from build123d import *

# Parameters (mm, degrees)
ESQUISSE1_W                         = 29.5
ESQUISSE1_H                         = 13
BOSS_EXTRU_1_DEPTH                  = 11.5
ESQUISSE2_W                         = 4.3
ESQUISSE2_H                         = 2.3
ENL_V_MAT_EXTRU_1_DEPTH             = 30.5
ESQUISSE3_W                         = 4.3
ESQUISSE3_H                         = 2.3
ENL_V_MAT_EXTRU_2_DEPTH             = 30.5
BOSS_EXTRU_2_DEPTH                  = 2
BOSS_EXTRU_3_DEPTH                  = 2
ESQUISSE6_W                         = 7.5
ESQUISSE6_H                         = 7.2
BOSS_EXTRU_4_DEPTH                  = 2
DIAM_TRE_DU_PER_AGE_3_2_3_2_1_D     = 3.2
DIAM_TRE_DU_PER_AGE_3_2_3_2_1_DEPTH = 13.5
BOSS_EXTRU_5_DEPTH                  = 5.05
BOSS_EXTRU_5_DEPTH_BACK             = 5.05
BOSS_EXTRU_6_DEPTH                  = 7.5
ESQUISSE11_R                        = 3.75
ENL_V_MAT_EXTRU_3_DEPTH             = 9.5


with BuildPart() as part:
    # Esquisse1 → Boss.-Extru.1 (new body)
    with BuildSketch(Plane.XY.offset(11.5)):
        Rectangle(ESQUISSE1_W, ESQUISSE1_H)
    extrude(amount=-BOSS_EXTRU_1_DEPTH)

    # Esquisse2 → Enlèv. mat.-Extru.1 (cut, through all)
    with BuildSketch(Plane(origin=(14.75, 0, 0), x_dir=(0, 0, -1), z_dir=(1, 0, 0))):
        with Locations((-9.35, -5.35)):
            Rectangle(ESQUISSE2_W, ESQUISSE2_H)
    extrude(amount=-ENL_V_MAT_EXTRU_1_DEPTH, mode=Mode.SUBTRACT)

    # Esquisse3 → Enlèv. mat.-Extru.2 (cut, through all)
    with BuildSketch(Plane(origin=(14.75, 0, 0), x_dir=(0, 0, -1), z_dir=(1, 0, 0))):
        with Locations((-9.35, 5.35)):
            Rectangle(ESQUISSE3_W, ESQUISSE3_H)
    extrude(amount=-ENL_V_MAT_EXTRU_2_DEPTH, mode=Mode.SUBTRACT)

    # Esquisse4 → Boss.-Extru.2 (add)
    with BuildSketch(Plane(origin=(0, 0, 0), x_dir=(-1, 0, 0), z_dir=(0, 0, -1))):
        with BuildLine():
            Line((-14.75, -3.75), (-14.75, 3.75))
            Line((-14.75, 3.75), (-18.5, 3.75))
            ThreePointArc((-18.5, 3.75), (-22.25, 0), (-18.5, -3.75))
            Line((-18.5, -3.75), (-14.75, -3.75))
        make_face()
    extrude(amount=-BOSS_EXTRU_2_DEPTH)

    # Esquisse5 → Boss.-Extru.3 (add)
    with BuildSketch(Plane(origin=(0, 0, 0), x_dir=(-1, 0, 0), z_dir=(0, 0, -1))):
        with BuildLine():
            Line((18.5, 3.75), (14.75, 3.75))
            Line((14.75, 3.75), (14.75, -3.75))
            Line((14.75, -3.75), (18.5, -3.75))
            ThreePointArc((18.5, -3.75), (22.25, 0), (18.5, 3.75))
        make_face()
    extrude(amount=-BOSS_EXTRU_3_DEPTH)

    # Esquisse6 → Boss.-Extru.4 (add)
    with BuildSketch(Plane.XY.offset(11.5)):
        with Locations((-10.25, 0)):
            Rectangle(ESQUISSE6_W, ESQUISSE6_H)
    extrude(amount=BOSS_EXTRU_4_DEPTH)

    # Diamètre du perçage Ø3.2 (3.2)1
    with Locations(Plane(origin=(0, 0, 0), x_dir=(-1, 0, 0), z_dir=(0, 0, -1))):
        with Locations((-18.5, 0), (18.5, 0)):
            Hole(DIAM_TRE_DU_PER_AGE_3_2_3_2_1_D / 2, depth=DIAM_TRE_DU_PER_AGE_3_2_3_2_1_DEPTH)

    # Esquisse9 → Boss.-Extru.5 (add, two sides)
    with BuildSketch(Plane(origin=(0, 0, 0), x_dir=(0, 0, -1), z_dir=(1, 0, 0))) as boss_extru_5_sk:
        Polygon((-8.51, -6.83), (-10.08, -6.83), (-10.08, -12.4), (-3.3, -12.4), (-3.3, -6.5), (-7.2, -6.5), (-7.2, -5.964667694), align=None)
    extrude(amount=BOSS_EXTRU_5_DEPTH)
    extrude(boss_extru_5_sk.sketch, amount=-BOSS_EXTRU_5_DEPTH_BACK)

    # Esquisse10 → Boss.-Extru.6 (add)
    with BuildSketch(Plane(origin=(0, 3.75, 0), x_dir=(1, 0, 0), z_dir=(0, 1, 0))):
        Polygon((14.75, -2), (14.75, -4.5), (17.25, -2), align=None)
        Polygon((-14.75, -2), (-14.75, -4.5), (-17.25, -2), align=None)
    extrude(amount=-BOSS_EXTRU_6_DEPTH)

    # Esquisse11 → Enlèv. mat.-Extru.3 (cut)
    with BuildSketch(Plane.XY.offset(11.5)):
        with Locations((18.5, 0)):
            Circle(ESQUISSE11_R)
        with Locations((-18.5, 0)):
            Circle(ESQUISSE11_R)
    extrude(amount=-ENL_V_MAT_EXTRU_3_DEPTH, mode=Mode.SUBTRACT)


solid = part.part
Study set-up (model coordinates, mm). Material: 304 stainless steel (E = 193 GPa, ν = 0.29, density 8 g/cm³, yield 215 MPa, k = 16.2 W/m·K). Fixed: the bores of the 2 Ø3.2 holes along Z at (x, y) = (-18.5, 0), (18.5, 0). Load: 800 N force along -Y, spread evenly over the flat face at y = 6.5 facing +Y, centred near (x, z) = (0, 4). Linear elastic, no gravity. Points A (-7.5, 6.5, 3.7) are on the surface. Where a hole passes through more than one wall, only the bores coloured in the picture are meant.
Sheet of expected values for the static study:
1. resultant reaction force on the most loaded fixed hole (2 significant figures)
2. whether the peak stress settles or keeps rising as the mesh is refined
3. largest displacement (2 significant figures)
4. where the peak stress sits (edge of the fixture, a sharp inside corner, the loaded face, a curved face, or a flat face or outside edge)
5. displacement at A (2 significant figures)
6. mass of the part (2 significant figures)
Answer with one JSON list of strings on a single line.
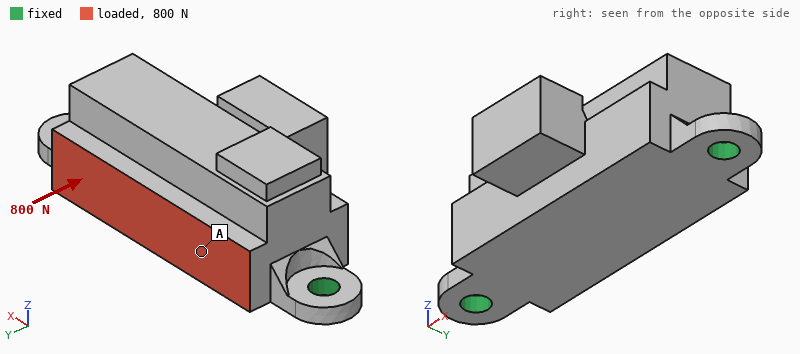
["400 N", "keeps rising", "21 µm", "edge of the fixture", "10 µm", "36 g"]
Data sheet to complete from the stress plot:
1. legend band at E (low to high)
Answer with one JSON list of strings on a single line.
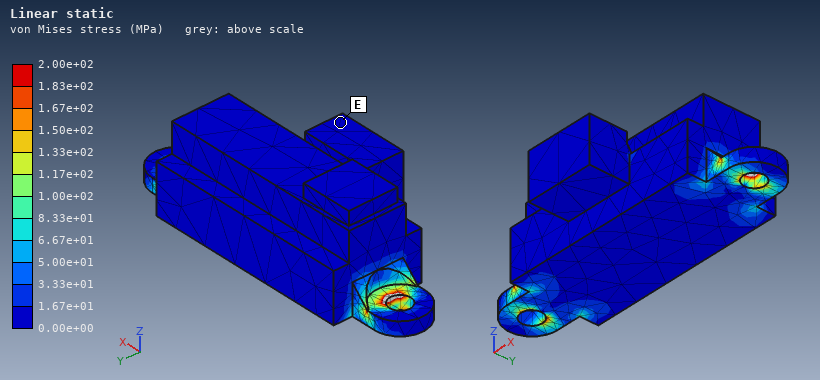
["0.00e+00 to 1.67e+01 MPa"]
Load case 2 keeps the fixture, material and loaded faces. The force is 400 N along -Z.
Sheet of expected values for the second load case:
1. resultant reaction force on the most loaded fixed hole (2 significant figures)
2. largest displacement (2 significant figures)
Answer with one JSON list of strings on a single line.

["250 N", "23 µm"]
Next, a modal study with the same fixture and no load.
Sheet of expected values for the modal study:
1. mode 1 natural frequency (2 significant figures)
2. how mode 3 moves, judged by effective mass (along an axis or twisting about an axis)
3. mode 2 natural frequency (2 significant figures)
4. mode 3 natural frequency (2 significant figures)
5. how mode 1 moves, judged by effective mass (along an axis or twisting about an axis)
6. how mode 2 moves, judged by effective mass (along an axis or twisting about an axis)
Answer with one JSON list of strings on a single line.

["4700 Hz", "along Y", "13 kHz", "18 kHz", "along Y", "along Z"]
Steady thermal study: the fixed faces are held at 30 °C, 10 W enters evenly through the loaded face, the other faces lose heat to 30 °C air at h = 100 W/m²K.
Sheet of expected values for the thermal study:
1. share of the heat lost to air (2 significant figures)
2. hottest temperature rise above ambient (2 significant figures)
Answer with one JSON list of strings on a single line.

["61 %", "52 K"]
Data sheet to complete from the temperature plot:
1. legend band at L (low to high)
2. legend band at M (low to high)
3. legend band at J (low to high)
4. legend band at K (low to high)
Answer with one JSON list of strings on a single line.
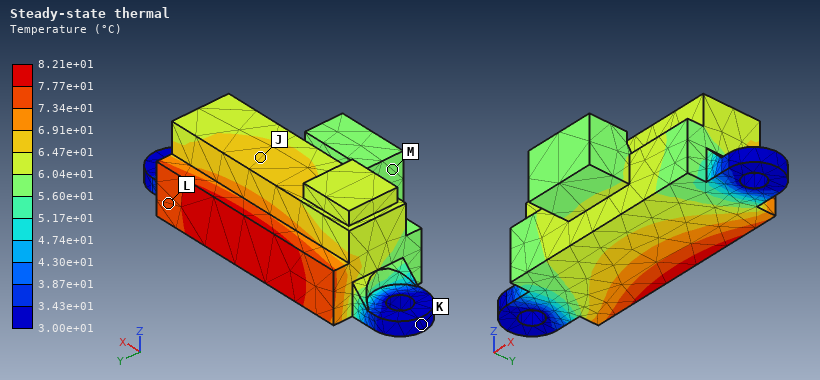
["7.34e+01 to 7.77e+01 °C", "5.60e+01 to 6.04e+01 °C", "6.47e+01 to 6.91e+01 °C", "3.00e+01 to 3.43e+01 °C"]
